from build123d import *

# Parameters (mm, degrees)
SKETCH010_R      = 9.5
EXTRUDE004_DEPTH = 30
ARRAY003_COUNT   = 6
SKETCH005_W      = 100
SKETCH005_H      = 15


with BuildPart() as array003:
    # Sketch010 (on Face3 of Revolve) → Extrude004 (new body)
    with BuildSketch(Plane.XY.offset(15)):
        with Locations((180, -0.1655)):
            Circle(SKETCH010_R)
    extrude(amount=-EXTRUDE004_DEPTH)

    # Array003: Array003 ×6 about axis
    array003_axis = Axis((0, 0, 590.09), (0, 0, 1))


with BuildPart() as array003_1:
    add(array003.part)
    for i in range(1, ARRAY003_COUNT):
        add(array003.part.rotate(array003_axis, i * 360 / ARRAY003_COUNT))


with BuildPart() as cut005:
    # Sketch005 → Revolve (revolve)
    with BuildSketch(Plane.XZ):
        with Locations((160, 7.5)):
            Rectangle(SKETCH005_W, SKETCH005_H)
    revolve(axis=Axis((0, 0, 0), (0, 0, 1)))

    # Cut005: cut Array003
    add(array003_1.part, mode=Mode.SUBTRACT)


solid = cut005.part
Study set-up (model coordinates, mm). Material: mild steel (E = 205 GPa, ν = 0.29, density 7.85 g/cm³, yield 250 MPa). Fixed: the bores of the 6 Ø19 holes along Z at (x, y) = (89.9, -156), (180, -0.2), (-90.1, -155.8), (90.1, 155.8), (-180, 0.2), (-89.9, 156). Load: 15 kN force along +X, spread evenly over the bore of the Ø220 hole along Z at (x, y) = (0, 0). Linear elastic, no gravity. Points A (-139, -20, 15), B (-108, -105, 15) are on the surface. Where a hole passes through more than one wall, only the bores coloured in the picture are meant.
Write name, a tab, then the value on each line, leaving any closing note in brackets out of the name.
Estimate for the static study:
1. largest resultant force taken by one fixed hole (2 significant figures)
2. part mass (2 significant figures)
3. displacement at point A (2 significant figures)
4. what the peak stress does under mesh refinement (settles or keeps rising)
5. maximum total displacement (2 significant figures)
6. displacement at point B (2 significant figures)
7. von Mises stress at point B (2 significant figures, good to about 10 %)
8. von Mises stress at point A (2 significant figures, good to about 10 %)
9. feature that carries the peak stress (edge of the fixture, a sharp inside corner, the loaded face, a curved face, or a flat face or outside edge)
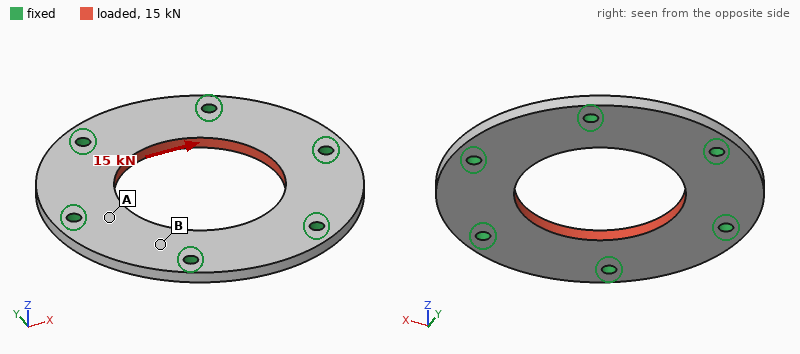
largest resultant force taken by one fixed hole	3.1 kN
part mass	12 kg
displacement at point A	0.67 µm
what the peak stress does under mesh refinement	keeps rising
maximum total displacement	1.3 µm
displacement at point B	0.83 µm
von Mises stress at point B	0.87 MPa
von Mises stress at point A	2.5 MPa
feature that carries the peak stress	edge of the fixture
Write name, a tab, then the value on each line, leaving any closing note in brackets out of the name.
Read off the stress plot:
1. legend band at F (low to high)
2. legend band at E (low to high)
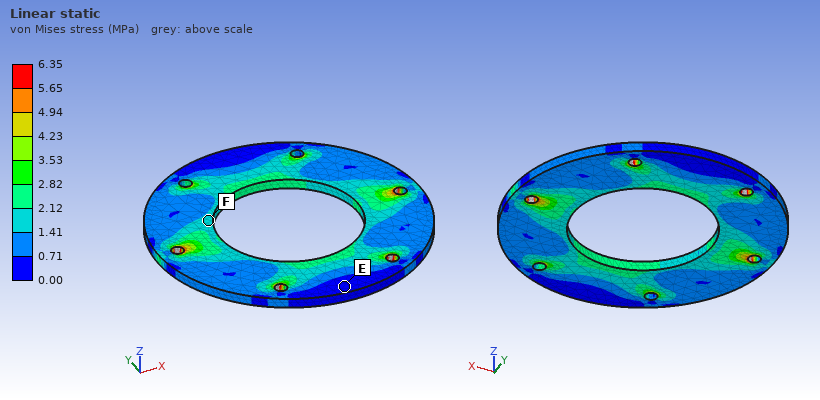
legend band at F	1.41 to 2.12 MPa
legend band at E	0.00 to 0.71 MPa
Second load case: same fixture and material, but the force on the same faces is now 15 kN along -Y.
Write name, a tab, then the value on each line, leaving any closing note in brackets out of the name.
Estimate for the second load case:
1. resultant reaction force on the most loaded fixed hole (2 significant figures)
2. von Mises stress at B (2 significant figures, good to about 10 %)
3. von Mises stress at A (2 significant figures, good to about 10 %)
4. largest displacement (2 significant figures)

resultant reaction force on the most loaded fixed hole	2.9 kN
von Mises stress at B	1.9 MPa
von Mises stress at A	1.2 MPa
largest displacement	1.3 µm
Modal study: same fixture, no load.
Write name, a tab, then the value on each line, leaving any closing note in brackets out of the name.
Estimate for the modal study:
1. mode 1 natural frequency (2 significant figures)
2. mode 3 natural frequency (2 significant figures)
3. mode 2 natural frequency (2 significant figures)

mode 1 natural frequency	2100 Hz
mode 3 natural frequency	2200 Hz
mode 2 natural frequency	2100 Hz
